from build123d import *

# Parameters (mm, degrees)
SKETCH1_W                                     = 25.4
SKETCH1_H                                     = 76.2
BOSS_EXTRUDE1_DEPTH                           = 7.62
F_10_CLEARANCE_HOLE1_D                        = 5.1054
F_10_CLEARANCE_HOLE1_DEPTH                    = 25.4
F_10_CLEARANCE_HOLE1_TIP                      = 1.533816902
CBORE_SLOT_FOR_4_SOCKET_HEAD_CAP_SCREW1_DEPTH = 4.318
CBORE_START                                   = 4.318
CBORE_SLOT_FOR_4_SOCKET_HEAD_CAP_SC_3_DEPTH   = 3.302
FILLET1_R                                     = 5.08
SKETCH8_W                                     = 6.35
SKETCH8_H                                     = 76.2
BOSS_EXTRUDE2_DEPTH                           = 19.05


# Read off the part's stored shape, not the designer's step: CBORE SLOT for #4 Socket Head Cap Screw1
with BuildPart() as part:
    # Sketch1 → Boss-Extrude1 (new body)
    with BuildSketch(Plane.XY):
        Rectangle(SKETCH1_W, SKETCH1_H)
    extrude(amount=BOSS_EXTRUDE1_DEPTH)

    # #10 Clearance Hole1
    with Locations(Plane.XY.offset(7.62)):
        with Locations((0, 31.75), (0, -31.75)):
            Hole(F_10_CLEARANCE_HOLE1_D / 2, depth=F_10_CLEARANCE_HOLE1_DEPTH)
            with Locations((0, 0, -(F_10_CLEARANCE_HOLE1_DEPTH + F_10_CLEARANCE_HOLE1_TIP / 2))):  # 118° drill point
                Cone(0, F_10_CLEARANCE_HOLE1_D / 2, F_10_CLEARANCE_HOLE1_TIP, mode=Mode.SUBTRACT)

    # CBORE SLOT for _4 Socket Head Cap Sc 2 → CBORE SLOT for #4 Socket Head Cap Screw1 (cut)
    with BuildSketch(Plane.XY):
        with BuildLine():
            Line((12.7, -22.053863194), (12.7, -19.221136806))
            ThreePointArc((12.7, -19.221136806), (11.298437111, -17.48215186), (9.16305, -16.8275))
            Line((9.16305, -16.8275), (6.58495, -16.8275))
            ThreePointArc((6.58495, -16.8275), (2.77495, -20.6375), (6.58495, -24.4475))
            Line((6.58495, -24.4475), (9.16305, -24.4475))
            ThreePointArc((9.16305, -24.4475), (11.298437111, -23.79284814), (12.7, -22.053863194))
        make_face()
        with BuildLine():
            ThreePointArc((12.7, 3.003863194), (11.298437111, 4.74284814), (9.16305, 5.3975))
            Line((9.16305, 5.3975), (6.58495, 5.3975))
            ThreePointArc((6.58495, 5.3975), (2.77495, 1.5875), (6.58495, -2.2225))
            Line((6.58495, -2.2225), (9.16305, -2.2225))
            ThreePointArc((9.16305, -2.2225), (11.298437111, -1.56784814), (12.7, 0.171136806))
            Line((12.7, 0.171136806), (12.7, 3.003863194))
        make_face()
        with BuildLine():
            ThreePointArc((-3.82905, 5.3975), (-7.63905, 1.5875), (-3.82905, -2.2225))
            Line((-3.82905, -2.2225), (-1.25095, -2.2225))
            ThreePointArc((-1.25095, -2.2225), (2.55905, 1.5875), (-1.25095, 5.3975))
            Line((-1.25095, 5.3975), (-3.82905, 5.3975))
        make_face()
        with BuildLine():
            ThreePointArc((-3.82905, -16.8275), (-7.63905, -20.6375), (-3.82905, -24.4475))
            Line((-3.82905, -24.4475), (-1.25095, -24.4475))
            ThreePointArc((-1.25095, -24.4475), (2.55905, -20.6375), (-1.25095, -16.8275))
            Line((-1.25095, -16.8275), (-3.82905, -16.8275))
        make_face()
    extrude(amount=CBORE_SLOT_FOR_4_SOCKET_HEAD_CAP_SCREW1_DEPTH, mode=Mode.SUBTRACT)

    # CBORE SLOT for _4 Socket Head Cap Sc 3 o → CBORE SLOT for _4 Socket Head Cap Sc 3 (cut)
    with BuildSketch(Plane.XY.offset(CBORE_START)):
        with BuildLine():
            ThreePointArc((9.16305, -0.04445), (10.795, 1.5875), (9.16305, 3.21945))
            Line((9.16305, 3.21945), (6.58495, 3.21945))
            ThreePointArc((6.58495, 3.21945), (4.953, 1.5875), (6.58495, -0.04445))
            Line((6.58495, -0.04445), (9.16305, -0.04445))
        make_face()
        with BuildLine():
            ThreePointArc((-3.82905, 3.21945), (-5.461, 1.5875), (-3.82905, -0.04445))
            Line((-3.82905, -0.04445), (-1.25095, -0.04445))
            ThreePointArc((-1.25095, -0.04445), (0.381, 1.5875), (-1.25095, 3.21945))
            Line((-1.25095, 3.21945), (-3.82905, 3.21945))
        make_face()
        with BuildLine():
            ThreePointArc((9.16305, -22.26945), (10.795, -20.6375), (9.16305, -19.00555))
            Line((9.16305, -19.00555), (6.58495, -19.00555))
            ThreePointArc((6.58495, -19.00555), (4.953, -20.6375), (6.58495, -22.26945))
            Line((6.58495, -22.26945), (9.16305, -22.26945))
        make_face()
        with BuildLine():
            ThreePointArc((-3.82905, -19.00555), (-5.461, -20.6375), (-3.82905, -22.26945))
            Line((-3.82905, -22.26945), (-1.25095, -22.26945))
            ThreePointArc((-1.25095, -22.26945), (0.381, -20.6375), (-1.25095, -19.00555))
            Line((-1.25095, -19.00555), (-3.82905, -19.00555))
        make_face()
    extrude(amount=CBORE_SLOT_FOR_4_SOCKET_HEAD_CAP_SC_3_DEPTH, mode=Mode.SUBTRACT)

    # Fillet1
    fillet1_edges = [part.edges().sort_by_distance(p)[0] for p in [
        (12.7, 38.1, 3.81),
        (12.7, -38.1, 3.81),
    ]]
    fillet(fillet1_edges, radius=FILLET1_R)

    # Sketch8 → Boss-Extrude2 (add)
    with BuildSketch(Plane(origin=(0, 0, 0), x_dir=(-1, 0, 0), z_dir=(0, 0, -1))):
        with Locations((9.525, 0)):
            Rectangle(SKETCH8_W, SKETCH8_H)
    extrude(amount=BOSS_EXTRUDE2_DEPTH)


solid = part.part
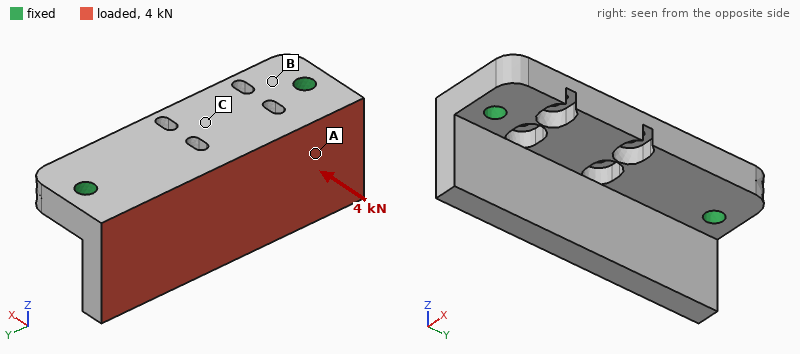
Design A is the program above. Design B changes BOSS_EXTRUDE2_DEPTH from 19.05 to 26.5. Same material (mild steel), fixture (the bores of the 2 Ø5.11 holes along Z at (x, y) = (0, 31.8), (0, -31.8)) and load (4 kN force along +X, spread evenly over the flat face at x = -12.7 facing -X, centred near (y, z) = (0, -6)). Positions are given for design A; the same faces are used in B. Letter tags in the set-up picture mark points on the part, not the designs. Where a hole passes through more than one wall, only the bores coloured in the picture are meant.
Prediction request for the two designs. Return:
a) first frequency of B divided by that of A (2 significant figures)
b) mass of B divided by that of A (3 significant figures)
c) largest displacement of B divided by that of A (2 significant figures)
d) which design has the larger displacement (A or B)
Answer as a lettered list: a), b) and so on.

a) 0.68
b) 1.16
c) 1.8
d) B
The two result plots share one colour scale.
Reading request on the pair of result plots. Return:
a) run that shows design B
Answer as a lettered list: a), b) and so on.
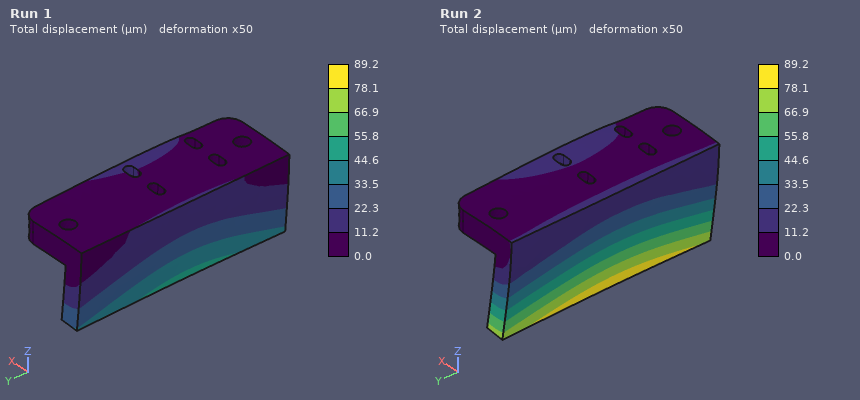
a) Run 2
